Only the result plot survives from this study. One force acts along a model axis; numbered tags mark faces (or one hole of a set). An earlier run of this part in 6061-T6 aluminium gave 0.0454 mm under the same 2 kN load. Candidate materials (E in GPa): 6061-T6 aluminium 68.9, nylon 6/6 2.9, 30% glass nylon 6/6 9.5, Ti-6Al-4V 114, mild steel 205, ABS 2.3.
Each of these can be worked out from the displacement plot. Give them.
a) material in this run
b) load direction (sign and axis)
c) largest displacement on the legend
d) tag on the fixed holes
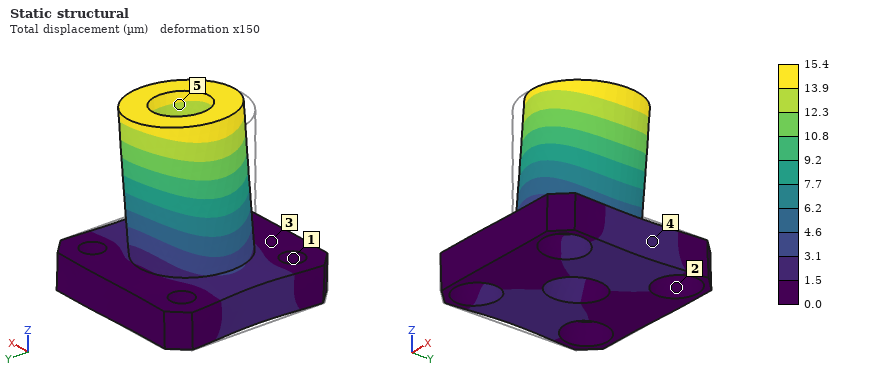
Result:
mild steel
+X
15.4 µm
1
